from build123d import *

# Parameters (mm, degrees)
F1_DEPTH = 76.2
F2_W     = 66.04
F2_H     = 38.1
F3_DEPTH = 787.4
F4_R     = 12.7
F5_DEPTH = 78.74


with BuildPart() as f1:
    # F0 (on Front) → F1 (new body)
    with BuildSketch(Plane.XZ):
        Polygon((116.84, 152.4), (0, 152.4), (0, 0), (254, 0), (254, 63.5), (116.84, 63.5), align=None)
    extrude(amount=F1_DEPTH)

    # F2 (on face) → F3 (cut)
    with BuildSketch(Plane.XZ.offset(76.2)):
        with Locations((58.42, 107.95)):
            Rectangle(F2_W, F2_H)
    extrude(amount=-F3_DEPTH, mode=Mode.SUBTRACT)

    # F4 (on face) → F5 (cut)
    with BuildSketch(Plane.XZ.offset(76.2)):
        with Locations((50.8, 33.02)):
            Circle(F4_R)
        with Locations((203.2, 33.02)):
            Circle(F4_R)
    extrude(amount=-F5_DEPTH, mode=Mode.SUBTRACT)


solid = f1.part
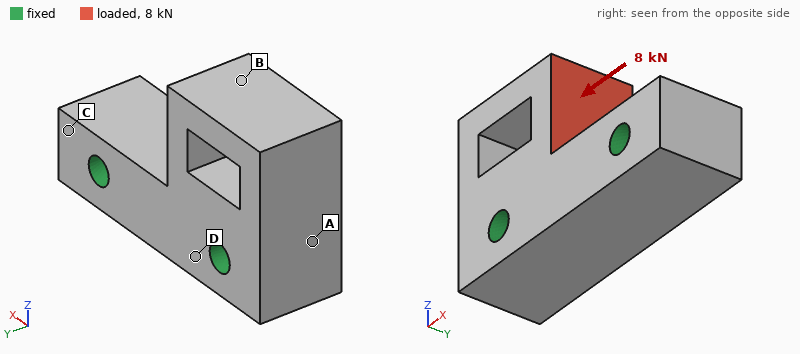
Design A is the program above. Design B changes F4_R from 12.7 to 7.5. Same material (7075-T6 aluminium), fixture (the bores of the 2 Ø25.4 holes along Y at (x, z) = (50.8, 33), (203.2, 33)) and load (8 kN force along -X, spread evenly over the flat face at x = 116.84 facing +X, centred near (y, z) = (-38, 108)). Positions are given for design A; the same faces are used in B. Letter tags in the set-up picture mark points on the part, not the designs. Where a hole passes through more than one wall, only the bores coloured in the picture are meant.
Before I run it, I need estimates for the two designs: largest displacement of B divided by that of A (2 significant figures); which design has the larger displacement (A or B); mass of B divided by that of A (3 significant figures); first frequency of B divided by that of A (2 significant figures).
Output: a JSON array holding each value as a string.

["1.2", "B", "1.03", "0.90"]
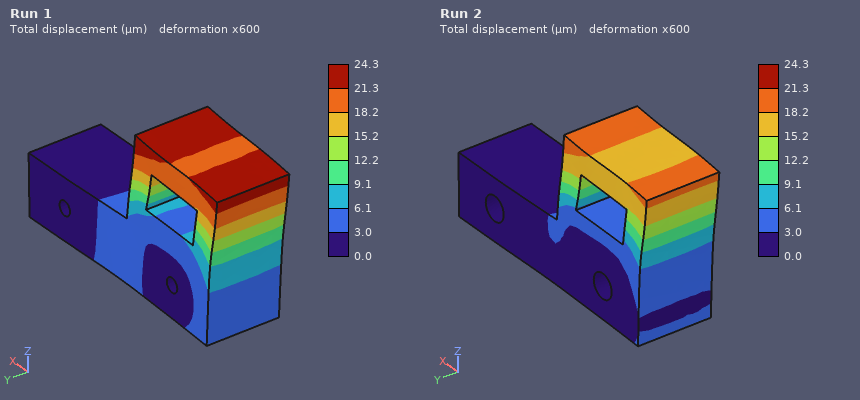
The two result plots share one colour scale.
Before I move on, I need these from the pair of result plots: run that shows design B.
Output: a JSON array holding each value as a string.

["Run 1"]
